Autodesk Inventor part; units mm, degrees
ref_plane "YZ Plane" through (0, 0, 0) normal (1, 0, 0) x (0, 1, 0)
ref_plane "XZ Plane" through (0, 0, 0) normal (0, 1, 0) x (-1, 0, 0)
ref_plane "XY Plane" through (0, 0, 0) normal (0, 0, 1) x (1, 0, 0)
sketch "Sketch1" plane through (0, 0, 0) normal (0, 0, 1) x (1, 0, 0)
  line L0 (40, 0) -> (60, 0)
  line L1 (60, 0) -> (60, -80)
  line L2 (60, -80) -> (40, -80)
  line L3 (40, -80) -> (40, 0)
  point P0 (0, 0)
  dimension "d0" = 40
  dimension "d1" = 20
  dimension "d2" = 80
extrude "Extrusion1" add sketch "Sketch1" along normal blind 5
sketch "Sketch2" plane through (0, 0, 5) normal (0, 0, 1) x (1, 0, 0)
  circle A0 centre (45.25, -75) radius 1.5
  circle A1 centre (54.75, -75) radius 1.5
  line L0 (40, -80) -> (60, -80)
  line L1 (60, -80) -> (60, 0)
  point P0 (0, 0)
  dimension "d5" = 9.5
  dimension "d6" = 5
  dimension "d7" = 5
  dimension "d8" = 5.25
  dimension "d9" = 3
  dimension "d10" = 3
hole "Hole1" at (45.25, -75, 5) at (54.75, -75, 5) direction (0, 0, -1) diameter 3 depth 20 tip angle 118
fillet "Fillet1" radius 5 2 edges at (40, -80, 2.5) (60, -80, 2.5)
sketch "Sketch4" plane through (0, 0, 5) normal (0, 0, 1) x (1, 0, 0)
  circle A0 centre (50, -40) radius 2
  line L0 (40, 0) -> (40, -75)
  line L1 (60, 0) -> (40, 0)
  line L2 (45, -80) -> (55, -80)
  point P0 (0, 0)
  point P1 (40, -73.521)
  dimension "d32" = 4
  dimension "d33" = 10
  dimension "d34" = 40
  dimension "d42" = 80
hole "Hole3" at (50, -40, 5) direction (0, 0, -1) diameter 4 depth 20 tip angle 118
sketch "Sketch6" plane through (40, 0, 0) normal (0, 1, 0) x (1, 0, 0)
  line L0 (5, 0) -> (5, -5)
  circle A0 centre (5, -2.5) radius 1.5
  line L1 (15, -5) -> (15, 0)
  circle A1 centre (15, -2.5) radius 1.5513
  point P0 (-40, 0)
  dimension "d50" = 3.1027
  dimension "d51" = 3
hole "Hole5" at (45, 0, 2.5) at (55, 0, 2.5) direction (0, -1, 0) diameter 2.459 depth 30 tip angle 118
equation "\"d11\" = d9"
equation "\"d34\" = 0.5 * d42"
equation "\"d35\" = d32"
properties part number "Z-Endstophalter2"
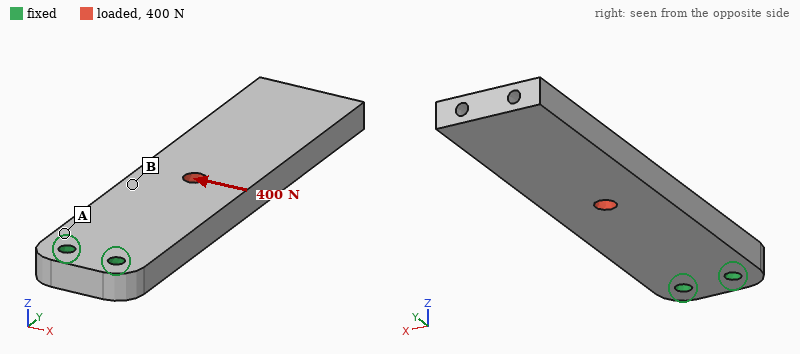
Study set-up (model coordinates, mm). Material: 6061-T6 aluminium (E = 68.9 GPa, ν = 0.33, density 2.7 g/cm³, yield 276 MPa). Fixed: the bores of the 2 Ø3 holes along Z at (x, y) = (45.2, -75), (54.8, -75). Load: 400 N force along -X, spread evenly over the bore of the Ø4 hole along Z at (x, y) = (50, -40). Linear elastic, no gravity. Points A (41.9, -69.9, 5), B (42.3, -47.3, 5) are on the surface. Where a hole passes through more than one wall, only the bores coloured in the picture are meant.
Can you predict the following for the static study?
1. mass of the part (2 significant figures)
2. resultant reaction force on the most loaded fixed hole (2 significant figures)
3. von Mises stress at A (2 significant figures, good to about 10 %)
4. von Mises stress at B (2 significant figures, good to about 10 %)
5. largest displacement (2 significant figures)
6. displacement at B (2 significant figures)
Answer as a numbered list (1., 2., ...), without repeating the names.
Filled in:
1. 20 g
2. 1.2 kN
3. 26 MPa
4. 8.1 MPa
5. 86 µm
6. 28 µm
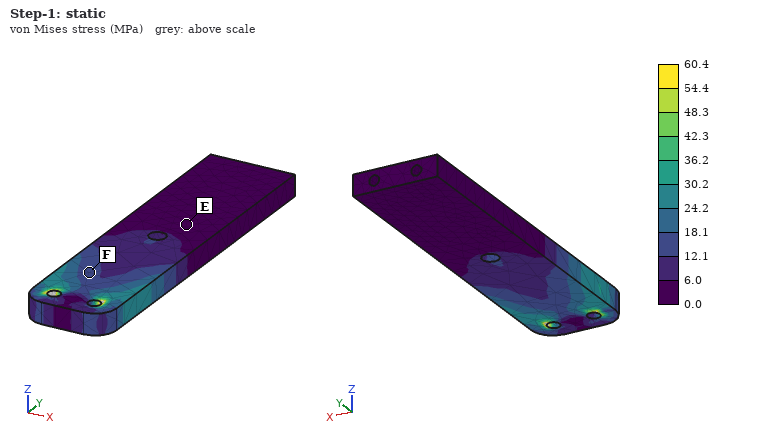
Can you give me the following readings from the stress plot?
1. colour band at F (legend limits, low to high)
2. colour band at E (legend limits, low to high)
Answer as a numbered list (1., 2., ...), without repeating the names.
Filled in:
1. 12.1 to 18.1 MPa
2. 0.0 to 6.0 MPa
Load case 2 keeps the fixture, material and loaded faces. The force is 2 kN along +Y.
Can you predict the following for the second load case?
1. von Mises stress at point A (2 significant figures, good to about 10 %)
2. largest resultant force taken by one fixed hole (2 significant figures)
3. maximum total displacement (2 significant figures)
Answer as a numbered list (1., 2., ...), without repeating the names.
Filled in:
1. 17 MPa
2. 1.0 kN
3. 13 µm
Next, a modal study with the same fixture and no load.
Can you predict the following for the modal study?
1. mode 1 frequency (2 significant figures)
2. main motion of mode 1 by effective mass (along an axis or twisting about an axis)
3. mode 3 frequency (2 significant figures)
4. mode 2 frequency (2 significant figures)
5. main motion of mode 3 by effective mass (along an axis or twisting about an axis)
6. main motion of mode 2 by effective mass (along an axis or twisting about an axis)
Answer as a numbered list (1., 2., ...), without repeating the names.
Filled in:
1. 760 Hz
2. along Z
3. 4500 Hz
4. 2700 Hz
5. along Z
6. along X
